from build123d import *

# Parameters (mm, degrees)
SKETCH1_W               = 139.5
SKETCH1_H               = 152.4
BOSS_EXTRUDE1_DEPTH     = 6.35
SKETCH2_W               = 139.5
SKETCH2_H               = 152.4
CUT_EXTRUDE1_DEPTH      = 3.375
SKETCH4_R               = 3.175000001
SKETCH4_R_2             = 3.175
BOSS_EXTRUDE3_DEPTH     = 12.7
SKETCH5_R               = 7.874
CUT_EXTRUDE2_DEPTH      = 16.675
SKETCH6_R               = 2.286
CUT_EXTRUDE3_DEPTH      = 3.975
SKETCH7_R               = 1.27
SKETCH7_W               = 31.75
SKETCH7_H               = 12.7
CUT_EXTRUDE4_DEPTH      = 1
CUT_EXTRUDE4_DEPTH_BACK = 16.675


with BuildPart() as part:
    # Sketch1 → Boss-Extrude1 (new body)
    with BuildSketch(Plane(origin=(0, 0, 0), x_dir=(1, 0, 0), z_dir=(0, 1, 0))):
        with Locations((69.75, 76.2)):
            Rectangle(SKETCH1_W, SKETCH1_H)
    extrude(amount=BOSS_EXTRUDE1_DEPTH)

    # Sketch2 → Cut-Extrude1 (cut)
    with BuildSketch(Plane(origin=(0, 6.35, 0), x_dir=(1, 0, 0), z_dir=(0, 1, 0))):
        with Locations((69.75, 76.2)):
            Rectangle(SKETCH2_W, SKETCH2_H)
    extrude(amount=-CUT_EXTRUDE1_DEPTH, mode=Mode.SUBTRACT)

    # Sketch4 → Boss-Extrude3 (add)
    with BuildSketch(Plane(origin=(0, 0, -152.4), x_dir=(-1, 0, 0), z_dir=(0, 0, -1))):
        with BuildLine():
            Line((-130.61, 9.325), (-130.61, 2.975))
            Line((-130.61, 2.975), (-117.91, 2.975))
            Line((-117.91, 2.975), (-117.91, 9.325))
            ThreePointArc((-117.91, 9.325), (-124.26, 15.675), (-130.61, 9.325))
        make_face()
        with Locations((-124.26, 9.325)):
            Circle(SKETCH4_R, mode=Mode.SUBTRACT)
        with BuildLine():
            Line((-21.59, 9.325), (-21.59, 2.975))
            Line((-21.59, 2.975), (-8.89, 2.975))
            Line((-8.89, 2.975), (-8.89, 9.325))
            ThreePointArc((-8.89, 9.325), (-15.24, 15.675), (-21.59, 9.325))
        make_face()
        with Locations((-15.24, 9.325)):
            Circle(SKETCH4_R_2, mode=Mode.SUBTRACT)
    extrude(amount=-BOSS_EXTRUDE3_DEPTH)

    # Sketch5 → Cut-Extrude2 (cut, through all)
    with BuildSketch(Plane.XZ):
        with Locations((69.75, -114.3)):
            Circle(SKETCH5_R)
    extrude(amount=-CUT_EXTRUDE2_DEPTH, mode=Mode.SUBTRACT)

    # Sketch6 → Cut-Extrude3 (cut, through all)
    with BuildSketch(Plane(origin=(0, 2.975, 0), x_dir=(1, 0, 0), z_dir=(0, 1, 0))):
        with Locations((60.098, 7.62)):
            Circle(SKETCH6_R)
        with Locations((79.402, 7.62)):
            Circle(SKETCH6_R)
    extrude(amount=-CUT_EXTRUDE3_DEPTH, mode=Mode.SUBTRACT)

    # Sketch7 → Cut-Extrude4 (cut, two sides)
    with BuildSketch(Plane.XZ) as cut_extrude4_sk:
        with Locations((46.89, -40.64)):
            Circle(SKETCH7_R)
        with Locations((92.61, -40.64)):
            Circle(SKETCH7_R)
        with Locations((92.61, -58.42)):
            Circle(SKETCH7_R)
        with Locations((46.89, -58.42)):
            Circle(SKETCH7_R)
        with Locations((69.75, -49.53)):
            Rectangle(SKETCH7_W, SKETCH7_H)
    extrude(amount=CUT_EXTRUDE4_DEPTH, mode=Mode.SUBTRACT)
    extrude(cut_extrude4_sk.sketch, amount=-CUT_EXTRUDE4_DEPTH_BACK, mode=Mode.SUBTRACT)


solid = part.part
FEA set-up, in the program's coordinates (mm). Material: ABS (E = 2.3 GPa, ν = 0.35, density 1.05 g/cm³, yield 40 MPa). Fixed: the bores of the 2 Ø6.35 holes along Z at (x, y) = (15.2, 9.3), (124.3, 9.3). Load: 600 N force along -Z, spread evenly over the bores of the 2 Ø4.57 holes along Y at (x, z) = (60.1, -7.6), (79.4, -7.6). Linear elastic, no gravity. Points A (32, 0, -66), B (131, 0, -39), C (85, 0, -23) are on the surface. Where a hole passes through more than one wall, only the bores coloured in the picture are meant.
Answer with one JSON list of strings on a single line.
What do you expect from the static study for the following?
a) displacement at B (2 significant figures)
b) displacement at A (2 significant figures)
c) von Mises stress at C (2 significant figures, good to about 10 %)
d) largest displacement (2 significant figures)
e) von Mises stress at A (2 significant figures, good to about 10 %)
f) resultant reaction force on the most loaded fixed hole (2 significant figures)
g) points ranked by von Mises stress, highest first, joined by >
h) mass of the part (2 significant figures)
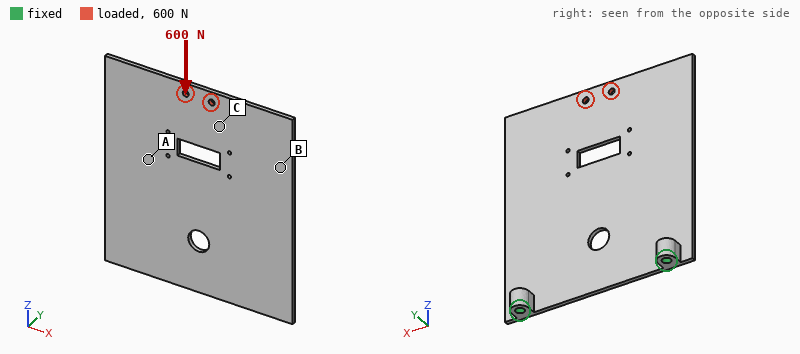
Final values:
["0.31 mm", "0.25 mm", "4.9 MPa", "0.48 mm", "2.6 MPa", "310 N", "C > A > B", "67 g"]
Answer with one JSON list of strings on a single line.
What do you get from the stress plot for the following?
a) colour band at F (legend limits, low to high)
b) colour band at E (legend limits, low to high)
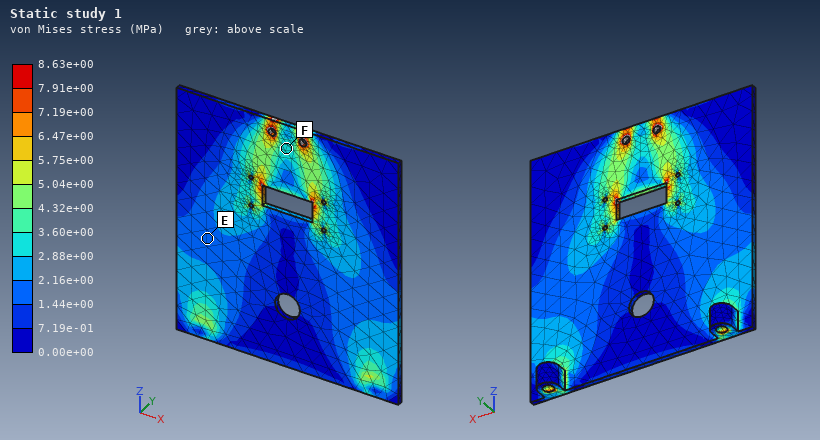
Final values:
["2.88e+00 to 3.60e+00 MPa", "1.44e+00 to 2.16e+00 MPa"]
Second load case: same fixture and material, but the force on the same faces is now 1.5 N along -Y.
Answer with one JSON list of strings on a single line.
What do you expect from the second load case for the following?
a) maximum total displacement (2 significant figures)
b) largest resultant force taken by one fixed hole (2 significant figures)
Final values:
["2.4 mm", "0.78 N"]
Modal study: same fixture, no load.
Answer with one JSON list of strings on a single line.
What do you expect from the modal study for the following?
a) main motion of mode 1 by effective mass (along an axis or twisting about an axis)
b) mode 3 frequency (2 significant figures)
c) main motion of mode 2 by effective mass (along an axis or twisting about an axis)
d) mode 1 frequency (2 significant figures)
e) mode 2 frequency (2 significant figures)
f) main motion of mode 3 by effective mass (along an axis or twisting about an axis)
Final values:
["along Y", "200 Hz", "twisting about Z", "31 Hz", "86 Hz", "along Y"]
